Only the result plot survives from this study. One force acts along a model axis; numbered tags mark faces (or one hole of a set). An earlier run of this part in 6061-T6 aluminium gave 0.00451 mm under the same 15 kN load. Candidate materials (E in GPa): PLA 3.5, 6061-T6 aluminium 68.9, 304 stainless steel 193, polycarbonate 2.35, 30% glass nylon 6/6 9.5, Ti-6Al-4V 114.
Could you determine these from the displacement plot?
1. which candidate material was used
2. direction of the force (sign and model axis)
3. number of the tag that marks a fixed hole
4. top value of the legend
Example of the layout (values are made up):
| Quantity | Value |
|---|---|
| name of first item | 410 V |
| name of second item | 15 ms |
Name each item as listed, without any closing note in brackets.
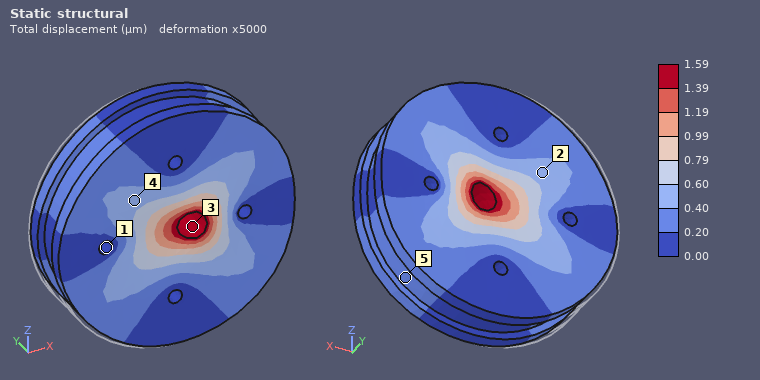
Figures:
| Quantity | Value |
|---|---|
| which candidate material was used | 304 stainless steel |
| direction of the force | +X |
| number of the tag that marks a fixed hole | 1 |
| top value of the legend | 1.59 µm |
